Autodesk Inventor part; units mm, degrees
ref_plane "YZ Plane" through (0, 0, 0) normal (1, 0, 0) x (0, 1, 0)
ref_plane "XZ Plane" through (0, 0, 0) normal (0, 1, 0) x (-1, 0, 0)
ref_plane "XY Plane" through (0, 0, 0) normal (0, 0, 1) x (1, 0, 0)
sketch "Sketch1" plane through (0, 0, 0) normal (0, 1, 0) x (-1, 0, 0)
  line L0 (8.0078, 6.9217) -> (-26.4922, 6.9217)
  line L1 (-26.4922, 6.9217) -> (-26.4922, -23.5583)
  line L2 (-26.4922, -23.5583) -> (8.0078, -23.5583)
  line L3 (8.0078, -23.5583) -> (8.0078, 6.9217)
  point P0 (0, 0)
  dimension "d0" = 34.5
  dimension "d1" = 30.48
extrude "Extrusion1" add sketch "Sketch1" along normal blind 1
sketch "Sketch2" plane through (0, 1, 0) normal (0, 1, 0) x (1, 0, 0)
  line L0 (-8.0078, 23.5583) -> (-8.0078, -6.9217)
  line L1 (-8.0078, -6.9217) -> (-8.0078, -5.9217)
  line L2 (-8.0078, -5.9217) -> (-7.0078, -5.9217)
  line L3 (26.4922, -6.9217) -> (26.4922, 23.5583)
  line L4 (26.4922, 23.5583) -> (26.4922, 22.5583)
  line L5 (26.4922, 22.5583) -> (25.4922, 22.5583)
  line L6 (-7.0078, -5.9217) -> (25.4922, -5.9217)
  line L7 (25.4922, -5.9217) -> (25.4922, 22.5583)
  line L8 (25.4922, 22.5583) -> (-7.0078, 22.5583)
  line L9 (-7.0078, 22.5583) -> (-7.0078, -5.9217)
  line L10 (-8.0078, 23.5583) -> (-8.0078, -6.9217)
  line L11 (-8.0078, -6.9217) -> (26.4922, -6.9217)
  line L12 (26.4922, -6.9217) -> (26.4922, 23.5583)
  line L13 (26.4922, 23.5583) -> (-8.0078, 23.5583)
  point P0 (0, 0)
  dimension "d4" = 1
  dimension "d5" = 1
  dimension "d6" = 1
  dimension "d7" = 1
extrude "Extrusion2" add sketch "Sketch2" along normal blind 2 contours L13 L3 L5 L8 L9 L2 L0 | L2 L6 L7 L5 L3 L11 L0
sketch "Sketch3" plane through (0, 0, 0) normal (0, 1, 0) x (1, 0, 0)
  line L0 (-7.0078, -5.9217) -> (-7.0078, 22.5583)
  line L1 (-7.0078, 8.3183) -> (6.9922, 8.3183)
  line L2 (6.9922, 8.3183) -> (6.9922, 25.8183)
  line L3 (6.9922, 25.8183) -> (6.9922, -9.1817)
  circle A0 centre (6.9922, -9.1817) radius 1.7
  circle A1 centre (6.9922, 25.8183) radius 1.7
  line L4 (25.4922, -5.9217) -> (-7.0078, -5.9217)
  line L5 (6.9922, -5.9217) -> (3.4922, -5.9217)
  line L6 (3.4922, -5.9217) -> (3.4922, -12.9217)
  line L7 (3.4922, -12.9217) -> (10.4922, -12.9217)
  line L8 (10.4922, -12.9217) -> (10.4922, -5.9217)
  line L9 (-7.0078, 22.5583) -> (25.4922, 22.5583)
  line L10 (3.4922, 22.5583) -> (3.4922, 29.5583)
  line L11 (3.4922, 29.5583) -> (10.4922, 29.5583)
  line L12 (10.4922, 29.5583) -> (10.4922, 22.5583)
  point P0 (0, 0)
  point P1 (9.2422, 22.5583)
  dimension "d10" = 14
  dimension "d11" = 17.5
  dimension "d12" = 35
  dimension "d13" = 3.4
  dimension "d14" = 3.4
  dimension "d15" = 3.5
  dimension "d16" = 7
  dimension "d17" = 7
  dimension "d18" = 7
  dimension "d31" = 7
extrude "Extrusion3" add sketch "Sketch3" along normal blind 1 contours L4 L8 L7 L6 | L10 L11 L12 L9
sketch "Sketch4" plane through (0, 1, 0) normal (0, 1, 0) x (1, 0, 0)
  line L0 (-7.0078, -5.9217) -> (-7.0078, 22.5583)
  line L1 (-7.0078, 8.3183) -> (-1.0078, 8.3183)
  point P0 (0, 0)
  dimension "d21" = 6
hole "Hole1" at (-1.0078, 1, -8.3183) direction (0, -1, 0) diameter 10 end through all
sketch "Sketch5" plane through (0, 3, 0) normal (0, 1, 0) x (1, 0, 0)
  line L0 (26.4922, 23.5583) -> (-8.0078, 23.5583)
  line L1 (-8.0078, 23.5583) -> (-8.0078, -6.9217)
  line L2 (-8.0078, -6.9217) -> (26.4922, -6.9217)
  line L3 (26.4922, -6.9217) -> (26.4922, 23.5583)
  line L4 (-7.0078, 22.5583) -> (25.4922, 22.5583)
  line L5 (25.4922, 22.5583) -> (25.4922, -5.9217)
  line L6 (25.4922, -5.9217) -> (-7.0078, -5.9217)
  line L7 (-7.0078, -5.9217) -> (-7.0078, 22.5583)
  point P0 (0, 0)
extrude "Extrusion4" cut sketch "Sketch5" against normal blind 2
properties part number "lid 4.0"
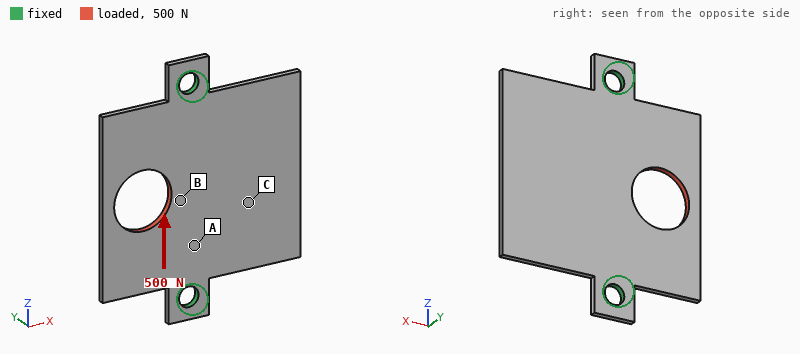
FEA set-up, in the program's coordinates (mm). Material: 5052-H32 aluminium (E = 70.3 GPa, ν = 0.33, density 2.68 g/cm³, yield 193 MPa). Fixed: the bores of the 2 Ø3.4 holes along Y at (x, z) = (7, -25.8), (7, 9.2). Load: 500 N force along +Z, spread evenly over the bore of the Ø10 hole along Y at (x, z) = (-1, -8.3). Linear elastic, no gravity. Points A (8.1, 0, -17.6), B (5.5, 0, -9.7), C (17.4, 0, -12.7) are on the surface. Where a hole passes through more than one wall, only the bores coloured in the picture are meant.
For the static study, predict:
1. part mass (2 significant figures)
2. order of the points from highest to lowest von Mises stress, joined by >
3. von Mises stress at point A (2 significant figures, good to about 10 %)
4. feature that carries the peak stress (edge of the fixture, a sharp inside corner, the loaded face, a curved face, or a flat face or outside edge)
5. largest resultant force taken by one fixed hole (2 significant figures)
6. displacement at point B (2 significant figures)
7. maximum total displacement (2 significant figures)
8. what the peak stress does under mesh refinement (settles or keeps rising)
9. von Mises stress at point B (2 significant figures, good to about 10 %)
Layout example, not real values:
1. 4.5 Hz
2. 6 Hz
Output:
1. 2.8 g
2. B > A > C
3. 17 MPa
4. a sharp inside corner
5. 280 N
6. 4.5 µm
7. 17 µm
8. keeps rising
9. 31 MPa
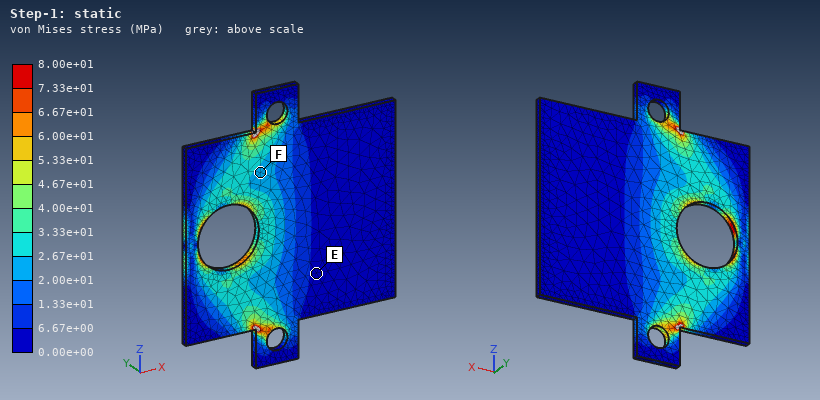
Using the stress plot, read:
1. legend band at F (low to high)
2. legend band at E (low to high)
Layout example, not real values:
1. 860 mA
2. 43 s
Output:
1. 2.00e+01 to 2.67e+01 MPa
2. 0.00e+00 to 6.67e+00 MPa
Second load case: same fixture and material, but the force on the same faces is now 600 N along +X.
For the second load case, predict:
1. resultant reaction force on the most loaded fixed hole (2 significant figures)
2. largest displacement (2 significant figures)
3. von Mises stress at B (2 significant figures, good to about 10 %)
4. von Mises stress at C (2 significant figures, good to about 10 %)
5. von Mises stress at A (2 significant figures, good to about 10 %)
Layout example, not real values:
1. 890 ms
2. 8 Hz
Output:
1. 300 N
2. 21 µm
3. 19 MPa
4. 14 MPa
5. 15 MPa
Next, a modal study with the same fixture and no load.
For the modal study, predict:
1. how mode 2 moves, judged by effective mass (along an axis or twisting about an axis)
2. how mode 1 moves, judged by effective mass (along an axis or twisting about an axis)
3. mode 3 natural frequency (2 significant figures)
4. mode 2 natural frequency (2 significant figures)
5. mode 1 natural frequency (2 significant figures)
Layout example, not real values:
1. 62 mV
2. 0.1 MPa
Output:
1. along Y
2. along Y
3. 3900 Hz
4. 2700 Hz
5. 1500 Hz
